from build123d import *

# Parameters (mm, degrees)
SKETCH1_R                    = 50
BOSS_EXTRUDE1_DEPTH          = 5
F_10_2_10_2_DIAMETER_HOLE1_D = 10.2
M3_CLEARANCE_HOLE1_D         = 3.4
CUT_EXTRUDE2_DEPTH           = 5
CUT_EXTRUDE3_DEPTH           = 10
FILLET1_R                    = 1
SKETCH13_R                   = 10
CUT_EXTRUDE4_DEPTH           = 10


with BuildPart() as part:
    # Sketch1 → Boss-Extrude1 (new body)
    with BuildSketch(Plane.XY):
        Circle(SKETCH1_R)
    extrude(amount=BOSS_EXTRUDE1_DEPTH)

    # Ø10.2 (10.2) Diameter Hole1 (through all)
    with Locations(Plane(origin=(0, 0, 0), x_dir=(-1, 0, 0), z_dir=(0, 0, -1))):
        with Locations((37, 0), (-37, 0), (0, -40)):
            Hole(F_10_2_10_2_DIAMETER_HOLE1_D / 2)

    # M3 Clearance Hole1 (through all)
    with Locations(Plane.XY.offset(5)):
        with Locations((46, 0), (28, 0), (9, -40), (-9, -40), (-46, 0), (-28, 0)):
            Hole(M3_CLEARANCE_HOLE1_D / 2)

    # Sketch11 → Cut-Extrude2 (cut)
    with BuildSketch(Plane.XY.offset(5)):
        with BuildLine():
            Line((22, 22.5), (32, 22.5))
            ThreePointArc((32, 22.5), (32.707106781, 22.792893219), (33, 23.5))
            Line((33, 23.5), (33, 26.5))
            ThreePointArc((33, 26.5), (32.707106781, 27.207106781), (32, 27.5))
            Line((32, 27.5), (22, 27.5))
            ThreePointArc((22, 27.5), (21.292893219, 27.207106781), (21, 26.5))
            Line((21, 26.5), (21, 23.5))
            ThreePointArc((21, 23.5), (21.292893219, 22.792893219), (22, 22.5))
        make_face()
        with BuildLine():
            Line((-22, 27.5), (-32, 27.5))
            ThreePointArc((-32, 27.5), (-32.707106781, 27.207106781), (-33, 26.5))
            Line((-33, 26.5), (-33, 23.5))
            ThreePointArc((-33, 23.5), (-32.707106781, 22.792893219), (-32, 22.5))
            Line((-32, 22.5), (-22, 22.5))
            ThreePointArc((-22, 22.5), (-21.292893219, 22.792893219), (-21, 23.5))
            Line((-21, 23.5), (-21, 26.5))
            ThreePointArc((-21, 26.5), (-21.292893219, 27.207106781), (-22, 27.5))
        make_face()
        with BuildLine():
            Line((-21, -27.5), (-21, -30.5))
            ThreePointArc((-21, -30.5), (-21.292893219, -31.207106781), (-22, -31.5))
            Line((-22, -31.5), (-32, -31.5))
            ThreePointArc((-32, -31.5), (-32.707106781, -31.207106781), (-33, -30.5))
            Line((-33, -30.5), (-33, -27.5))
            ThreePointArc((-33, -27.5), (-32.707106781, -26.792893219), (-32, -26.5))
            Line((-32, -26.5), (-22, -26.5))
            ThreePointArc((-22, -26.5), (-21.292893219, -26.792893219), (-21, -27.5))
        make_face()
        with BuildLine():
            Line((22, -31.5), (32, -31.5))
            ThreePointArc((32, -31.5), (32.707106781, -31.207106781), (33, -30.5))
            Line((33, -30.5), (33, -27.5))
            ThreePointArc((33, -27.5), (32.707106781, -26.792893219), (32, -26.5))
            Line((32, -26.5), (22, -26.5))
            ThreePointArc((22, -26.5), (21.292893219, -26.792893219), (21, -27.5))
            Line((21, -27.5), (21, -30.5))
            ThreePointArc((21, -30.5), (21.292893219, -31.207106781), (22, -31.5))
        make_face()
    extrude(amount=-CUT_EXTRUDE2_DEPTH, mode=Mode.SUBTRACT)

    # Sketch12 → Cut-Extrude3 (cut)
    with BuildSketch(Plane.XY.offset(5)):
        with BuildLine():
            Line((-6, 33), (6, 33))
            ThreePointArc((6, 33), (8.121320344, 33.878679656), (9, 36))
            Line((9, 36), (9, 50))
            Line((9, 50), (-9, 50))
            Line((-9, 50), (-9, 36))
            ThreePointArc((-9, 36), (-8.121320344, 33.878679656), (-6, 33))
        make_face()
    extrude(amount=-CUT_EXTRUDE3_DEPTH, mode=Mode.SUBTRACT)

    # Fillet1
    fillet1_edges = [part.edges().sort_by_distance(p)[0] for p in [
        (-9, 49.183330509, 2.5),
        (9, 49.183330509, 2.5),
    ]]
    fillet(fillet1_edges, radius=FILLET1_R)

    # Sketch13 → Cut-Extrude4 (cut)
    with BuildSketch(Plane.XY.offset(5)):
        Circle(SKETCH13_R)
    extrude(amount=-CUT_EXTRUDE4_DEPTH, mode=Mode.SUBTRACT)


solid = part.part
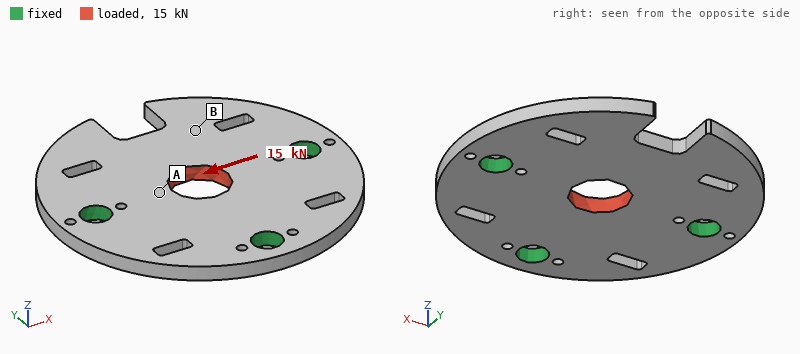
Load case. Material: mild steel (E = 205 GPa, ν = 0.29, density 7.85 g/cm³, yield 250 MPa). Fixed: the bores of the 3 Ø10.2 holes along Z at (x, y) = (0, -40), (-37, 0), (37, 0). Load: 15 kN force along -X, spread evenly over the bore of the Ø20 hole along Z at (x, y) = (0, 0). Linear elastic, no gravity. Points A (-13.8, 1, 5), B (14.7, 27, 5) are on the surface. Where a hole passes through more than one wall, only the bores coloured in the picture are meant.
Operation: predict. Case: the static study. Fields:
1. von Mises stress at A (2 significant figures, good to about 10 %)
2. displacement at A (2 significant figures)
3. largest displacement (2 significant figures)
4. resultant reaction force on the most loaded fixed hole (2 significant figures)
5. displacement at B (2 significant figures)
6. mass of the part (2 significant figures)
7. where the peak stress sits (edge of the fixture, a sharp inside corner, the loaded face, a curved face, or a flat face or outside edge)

53 MPa
5.9 µm
8.7 µm
6.5 kN
5.0 µm
260 g
a curved face
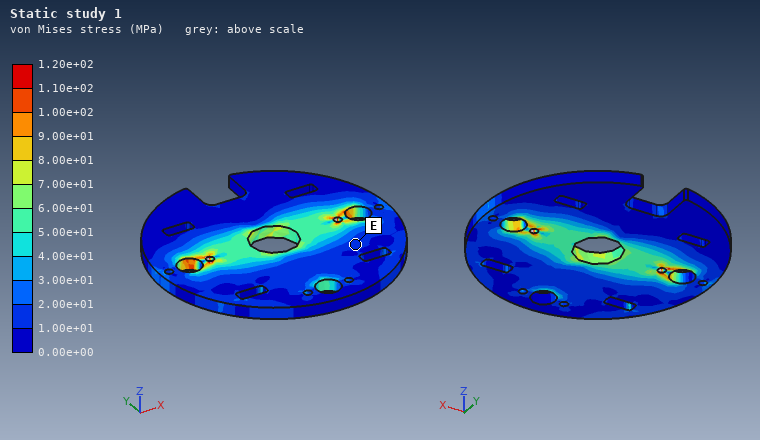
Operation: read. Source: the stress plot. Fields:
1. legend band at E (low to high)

1.00e+01 to 2.00e+01 MPa
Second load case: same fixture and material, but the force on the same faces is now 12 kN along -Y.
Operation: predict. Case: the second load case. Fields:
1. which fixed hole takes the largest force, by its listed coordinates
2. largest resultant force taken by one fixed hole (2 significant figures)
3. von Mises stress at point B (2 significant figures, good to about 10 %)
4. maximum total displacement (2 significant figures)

(0, -40)
5.0 kN
24 MPa
10 µm
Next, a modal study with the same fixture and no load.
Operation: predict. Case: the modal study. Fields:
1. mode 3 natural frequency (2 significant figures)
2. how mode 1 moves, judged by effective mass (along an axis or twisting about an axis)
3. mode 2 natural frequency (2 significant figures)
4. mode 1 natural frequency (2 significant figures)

6400 Hz
along Z
4000 Hz
2200 Hz
